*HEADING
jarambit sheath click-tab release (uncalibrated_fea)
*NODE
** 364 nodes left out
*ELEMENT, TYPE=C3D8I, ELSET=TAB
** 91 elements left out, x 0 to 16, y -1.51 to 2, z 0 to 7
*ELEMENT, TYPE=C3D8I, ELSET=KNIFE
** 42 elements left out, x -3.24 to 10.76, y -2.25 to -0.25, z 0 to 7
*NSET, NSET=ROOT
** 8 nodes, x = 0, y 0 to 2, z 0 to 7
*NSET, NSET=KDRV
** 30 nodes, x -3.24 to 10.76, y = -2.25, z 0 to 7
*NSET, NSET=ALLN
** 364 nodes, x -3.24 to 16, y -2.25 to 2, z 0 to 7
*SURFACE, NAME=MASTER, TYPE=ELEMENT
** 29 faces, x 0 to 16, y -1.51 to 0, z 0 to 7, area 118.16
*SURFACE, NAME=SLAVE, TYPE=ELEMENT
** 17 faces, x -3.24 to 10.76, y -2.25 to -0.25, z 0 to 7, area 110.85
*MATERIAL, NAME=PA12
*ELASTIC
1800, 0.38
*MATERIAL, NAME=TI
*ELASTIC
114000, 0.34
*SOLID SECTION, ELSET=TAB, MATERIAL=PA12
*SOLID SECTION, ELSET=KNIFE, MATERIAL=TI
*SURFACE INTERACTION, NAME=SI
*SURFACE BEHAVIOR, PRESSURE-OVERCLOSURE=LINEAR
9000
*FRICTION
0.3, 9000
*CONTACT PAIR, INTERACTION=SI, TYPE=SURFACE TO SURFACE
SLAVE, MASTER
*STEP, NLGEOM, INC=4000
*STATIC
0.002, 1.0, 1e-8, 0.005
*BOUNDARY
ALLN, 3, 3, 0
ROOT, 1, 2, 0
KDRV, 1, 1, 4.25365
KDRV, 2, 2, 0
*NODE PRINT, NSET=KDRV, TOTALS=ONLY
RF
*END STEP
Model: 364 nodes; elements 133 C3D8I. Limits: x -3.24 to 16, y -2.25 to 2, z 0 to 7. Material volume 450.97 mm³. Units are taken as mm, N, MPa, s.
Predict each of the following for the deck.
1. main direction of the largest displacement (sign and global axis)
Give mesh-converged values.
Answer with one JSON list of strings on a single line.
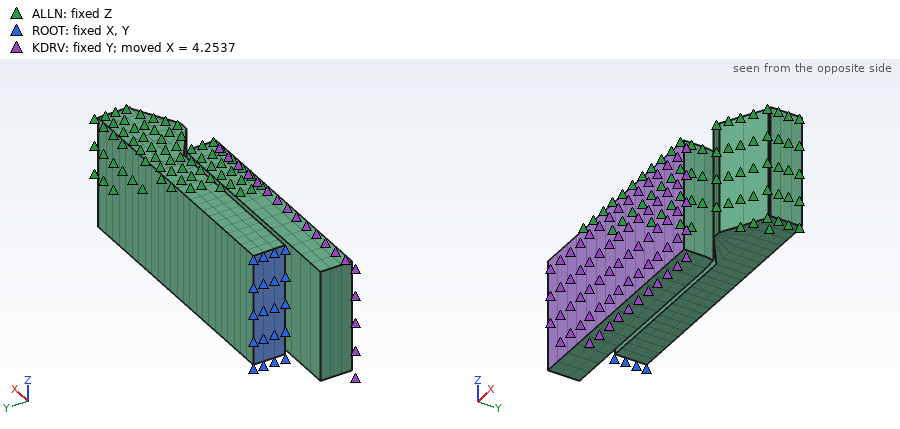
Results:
["+X"]
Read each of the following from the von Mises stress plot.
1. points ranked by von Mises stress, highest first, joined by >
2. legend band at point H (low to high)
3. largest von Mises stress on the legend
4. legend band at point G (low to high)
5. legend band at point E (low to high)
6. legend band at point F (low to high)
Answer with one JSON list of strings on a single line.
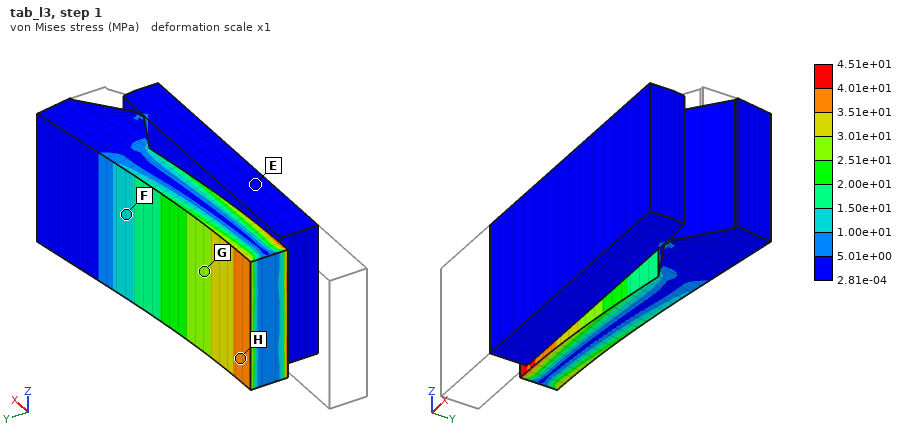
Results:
["H > G > F > E", "3.51e+01 to 4.01e+01 MPa", "4.51e+01 MPa", "2.51e+01 to 3.01e+01 MPa", "2.81e-04 to 5.01e+00 MPa", "1.00e+01 to 1.50e+01 MPa"]
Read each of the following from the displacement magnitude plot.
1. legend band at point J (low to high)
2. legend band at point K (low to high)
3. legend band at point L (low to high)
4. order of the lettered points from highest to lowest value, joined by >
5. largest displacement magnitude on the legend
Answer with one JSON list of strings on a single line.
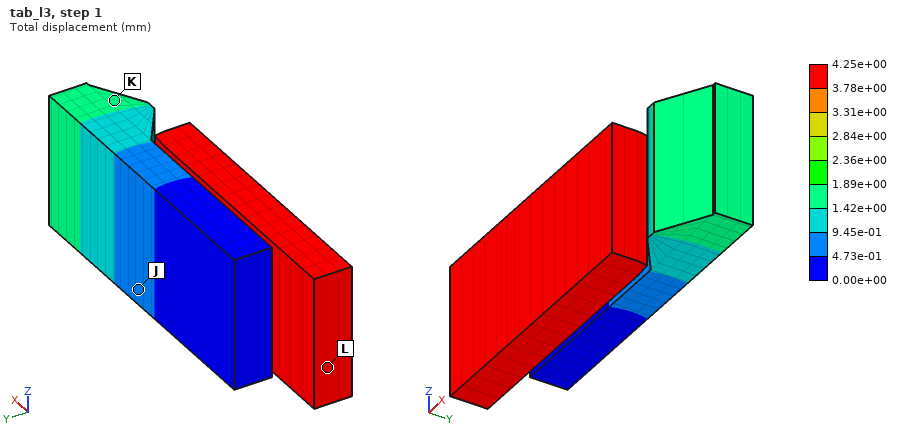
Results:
["4.73e-01 to 9.45e-01 mm", "1.42e+00 to 1.89e+00 mm", "3.78e+00 to 4.25e+00 mm", "L > K > J", "4.25e+00 mm"]
